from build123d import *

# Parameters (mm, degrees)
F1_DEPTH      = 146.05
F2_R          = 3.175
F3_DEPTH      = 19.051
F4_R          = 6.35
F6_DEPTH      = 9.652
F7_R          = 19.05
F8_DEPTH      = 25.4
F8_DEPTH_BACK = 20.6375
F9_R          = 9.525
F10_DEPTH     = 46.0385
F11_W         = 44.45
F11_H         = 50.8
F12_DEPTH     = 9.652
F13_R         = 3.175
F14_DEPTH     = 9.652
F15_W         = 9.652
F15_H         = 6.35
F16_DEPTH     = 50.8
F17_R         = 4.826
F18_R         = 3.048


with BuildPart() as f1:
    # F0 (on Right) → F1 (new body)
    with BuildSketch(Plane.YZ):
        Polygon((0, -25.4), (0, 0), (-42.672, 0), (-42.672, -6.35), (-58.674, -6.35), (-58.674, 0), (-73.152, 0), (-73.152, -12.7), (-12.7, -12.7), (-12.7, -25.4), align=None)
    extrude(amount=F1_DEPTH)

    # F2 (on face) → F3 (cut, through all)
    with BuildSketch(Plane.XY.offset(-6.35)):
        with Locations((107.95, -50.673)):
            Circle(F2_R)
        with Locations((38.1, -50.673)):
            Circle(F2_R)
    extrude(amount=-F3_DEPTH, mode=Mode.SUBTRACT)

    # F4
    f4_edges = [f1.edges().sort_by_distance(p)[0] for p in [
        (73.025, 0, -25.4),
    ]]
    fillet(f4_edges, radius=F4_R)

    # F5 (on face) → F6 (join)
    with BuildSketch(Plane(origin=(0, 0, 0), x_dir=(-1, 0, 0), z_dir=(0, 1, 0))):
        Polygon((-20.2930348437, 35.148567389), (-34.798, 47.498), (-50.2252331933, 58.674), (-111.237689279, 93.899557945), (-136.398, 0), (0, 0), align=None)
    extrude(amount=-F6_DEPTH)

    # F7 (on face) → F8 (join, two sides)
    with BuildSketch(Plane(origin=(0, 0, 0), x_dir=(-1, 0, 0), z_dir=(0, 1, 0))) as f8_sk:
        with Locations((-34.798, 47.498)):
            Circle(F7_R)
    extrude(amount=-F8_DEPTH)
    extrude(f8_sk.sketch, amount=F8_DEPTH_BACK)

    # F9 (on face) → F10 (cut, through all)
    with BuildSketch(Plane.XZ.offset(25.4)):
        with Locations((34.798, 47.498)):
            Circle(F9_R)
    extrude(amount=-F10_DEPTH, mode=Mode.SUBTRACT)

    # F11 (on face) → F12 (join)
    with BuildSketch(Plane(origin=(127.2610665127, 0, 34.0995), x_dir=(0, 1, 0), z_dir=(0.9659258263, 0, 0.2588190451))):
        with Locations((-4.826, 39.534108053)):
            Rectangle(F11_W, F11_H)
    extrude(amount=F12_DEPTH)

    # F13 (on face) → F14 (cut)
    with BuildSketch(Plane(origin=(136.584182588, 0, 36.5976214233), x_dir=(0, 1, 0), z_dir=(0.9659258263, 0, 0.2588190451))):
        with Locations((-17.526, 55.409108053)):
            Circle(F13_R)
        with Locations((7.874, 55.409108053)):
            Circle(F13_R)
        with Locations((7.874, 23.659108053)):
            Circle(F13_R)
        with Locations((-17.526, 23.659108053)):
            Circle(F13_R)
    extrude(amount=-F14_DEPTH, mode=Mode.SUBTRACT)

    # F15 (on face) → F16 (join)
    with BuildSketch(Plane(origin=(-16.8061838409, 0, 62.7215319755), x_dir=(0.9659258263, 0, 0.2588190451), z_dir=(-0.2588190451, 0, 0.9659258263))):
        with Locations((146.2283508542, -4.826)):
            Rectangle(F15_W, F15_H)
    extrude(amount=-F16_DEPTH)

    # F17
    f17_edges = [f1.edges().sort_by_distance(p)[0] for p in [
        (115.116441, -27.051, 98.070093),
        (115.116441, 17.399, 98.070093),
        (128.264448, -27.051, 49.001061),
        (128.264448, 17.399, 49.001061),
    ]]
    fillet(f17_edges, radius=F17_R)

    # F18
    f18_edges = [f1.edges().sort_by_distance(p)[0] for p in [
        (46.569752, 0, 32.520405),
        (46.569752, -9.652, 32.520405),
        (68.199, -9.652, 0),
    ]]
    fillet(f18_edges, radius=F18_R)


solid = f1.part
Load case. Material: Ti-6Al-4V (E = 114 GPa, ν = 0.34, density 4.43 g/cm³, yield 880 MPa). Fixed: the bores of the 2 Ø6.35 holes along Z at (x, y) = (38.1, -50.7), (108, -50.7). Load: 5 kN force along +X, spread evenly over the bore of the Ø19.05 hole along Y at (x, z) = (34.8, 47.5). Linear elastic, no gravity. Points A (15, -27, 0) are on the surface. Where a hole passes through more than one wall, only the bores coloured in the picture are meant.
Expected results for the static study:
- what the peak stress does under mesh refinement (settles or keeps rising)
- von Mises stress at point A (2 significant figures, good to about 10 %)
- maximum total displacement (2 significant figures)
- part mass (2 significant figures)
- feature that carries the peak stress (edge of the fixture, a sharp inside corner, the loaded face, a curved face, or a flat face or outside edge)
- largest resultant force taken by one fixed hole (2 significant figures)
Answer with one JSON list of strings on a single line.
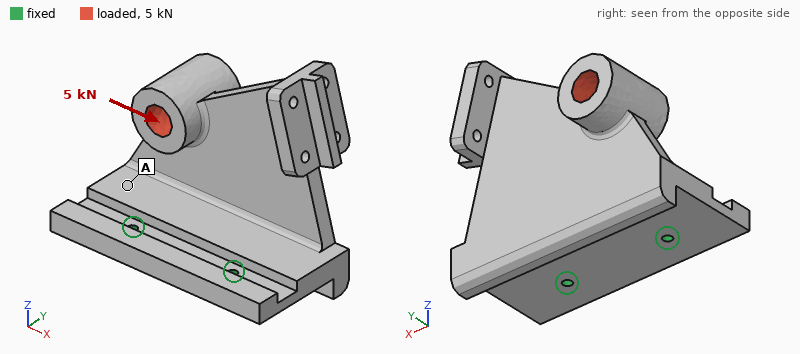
["keeps rising", "18 MPa", "0.29 mm", "1.2 kg", "edge of the fixture", "5.6 kN"]
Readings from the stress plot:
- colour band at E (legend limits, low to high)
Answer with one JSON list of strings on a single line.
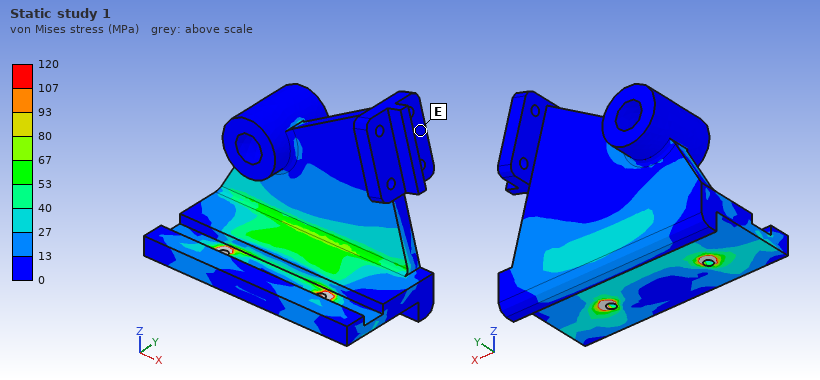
["0 to 13 MPa"]
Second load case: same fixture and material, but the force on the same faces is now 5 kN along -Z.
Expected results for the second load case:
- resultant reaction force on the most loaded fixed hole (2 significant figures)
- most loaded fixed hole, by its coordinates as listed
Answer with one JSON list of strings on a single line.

["5.0 kN", "(38.1, -50.7)"]
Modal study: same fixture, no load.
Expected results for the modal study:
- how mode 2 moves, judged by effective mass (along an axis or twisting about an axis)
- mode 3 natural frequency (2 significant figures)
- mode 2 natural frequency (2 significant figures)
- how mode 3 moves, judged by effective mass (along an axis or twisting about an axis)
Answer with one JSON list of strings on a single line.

["along X", "1200 Hz", "900 Hz", "along Z"]
